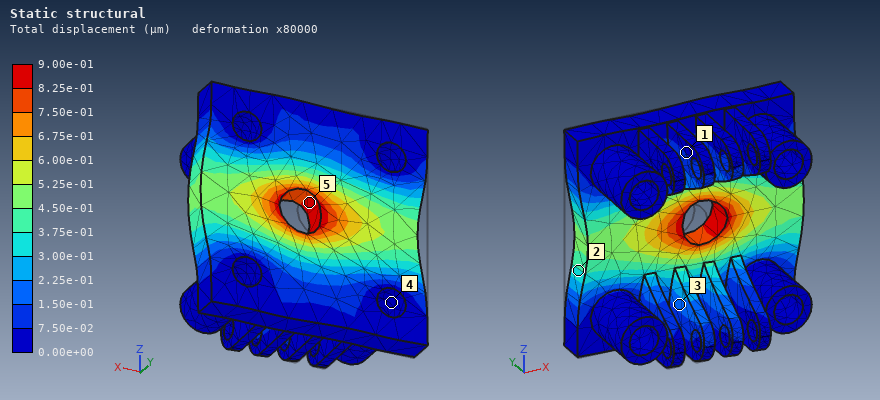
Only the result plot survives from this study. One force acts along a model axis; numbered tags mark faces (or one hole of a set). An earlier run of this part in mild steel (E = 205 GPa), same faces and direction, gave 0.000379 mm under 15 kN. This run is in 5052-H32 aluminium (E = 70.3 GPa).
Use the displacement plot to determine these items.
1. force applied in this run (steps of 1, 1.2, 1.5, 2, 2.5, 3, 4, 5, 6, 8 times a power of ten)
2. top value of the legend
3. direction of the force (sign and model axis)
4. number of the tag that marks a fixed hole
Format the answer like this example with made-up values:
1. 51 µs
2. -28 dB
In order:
1. 12 kN
2. 9.00e-01 µm
3. +X
4. 4
